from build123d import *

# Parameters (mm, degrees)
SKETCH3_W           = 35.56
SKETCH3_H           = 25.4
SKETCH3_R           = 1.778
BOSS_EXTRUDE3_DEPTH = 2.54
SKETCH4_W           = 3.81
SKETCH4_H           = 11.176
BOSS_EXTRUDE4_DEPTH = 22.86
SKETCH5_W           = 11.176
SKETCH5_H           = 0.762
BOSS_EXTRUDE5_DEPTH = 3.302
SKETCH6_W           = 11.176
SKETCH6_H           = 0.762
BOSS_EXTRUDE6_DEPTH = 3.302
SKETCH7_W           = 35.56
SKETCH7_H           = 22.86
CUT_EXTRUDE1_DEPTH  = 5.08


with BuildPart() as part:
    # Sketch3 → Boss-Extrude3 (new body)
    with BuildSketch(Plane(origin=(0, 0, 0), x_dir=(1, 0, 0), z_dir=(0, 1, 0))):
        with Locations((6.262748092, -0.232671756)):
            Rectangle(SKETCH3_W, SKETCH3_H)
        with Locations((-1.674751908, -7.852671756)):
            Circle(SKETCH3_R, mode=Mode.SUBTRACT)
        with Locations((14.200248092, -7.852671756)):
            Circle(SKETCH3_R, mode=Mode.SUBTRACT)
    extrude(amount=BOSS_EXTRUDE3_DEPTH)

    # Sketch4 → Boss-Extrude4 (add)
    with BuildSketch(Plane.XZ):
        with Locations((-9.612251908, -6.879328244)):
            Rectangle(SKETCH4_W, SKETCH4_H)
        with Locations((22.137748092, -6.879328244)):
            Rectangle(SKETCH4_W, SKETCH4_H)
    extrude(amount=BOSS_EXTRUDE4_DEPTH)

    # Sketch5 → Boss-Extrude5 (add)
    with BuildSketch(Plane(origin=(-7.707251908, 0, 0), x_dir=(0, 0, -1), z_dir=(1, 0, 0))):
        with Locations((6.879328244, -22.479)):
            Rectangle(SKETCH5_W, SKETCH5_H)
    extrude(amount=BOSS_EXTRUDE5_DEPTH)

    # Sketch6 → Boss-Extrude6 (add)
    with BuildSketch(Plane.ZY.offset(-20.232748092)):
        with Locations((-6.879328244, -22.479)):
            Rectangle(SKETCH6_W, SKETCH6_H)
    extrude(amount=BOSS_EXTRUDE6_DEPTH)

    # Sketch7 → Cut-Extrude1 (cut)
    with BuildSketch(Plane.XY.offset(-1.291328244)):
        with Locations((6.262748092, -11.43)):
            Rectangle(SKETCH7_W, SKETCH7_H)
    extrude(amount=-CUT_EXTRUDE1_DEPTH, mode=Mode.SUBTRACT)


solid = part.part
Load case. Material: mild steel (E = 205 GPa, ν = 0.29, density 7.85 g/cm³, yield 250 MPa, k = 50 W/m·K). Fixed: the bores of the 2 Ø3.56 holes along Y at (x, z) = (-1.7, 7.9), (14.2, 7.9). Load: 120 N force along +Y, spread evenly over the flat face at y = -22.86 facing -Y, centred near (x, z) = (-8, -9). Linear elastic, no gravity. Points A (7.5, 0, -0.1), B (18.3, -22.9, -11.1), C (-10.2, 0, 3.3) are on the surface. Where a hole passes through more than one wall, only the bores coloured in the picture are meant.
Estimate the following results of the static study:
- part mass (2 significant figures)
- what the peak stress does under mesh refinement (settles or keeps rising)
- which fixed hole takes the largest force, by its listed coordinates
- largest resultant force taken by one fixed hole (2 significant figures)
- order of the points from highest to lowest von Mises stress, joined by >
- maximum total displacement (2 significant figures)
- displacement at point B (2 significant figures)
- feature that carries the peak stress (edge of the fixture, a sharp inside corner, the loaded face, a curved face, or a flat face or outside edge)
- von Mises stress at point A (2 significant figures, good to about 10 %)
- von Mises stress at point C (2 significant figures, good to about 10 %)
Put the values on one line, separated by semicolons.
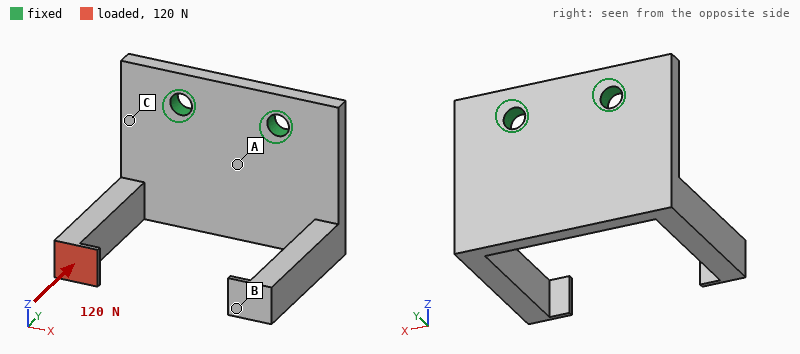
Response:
26 g; keeps rising; (-1.7, 7.9); 140 N; C > A > B; 91 µm; 24 µm; edge of the fixture; 33 MPa; 54 MPa
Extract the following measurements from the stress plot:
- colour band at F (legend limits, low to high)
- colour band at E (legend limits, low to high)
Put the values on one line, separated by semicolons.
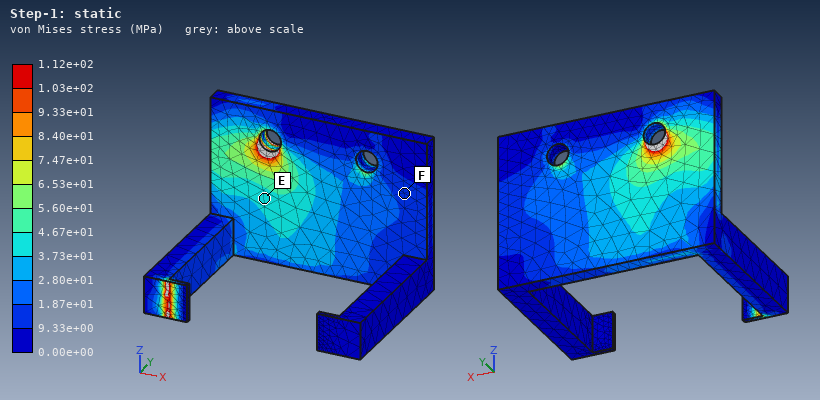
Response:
9.33e+00 to 1.87e+01 MPa; 3.73e+01 to 4.67e+01 MPa
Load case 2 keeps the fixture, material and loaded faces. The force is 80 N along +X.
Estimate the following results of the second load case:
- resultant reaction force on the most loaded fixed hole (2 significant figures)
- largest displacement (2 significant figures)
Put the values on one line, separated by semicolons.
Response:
110 N; 0.20 mm
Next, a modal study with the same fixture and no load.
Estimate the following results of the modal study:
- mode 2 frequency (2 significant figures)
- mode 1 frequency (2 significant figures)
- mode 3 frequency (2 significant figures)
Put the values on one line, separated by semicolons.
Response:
2200 Hz; 2100 Hz; 2700 Hz
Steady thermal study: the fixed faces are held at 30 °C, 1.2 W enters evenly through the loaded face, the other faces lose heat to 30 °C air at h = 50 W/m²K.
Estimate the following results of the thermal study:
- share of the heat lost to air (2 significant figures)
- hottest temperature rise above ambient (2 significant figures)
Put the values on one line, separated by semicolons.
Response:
46 %; 30 K
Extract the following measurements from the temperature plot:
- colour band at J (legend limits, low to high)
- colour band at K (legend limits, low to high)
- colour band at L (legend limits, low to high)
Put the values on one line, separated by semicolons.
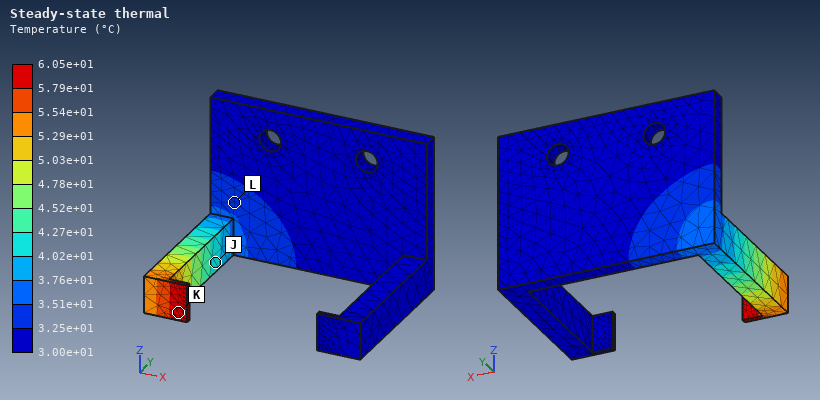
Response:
4.02e+01 to 4.27e+01 °C; 5.79e+01 to 6.05e+01 °C; 3.25e+01 to 3.51e+01 °C
